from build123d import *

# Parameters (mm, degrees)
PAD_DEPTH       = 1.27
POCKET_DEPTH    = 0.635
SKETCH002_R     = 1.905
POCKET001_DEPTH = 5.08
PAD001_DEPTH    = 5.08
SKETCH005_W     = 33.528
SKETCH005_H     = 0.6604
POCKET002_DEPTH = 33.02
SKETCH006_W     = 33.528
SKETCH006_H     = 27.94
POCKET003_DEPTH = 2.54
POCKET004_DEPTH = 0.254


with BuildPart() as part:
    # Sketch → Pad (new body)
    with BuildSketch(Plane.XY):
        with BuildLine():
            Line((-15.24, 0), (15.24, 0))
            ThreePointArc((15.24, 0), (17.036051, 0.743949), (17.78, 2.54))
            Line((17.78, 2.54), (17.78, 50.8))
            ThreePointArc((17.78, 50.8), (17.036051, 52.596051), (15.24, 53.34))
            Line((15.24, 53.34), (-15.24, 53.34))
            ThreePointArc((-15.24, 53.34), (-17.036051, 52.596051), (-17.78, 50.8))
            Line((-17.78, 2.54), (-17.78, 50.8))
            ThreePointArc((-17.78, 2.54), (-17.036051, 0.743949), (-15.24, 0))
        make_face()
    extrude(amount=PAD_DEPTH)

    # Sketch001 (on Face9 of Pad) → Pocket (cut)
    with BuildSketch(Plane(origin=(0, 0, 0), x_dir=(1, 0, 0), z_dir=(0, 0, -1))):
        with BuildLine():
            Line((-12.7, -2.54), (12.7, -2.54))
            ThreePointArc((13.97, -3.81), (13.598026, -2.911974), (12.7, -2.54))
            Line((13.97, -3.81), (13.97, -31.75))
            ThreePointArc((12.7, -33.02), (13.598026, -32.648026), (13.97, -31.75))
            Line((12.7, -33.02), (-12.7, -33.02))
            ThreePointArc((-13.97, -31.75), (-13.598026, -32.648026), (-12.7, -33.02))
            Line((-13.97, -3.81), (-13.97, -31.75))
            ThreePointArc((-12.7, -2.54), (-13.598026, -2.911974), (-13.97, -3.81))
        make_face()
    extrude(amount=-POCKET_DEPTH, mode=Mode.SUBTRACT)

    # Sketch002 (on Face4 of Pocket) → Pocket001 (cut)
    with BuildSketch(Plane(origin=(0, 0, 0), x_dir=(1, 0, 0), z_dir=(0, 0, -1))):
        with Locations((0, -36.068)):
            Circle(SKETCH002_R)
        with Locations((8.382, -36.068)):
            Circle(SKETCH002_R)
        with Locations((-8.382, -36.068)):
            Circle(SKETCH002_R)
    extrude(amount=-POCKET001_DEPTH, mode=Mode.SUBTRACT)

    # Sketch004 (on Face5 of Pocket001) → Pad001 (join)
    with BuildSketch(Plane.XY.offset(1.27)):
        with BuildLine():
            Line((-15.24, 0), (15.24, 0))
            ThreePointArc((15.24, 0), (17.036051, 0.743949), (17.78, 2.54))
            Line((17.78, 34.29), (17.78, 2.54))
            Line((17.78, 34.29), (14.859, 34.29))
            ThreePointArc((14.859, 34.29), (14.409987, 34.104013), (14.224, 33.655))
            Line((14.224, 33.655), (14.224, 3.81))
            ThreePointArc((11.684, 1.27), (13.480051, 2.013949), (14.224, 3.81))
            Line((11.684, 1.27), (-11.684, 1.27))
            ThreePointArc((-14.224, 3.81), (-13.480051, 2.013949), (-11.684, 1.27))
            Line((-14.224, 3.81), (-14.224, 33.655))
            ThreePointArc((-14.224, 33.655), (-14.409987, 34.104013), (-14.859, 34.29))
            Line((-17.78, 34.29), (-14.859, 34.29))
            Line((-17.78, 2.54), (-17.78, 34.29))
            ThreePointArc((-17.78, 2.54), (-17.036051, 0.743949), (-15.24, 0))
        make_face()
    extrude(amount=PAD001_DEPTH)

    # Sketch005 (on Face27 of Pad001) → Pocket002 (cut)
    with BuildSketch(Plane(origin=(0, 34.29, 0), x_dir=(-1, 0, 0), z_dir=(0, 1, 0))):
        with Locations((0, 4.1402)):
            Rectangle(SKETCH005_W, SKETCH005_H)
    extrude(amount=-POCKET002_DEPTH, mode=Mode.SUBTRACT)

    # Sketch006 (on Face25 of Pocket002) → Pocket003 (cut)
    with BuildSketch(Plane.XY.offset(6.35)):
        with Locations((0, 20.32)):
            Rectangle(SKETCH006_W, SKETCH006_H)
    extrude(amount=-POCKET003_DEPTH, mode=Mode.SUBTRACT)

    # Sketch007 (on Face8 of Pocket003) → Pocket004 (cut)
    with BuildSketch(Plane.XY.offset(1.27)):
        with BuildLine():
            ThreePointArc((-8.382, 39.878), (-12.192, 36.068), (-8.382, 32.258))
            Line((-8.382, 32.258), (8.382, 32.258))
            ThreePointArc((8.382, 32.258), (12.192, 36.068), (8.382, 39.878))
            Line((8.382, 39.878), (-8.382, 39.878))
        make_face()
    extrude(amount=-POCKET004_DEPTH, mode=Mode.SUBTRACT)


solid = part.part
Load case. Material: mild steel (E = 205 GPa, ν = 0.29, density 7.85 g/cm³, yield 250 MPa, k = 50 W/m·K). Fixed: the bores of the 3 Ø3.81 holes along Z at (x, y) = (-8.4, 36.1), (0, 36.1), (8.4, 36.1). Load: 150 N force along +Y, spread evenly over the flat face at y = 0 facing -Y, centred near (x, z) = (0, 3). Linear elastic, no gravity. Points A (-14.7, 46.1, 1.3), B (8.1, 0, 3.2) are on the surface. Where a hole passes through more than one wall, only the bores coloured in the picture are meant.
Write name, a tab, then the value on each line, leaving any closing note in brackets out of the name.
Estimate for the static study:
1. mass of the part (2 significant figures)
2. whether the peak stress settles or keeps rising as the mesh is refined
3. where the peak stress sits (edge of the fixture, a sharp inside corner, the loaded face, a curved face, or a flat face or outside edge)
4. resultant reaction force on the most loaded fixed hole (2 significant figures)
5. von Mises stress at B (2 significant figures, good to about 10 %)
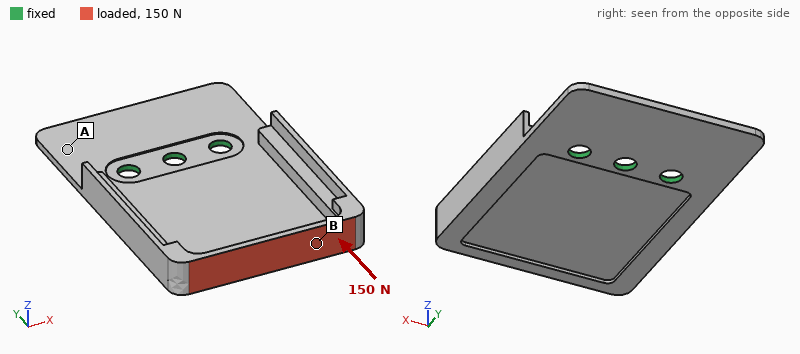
mass of the part	22 g
whether the peak stress settles or keeps rising as the mesh is refined	keeps rising
where the peak stress sits	a sharp inside corner
resultant reaction force on the most loaded fixed hole	52 N
von Mises stress at B	28 MPa
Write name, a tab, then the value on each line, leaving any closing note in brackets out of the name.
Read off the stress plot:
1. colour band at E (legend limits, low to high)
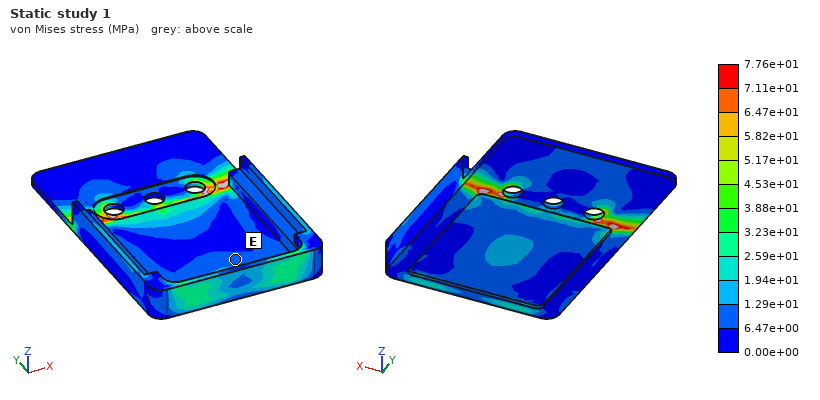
colour band at E	6.47e+00 to 1.29e+01 MPa
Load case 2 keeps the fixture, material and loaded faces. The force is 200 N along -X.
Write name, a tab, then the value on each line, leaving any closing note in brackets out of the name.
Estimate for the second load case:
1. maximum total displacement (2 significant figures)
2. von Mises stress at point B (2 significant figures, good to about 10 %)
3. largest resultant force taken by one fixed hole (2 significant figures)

maximum total displacement	84 µm
von Mises stress at point B	26 MPa
largest resultant force taken by one fixed hole	360 N
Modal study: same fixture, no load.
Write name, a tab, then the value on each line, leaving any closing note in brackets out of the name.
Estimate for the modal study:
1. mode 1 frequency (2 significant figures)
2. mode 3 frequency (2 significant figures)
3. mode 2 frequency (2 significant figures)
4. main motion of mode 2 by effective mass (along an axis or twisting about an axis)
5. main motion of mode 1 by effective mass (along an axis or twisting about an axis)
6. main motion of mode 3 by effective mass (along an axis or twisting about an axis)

mode 1 frequency	600 Hz
mode 3 frequency	3500 Hz
mode 2 frequency	1300 Hz
main motion of mode 2 by effective mass	twisting about Y
main motion of mode 1 by effective mass	along Z
main motion of mode 3 by effective mass	along Z
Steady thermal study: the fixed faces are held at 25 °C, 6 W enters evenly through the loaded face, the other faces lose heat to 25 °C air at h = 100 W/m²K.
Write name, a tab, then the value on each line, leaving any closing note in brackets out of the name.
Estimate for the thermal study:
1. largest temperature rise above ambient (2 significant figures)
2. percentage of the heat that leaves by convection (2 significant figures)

largest temperature rise above ambient	43 K
percentage of the heat that leaves by convection	87 %
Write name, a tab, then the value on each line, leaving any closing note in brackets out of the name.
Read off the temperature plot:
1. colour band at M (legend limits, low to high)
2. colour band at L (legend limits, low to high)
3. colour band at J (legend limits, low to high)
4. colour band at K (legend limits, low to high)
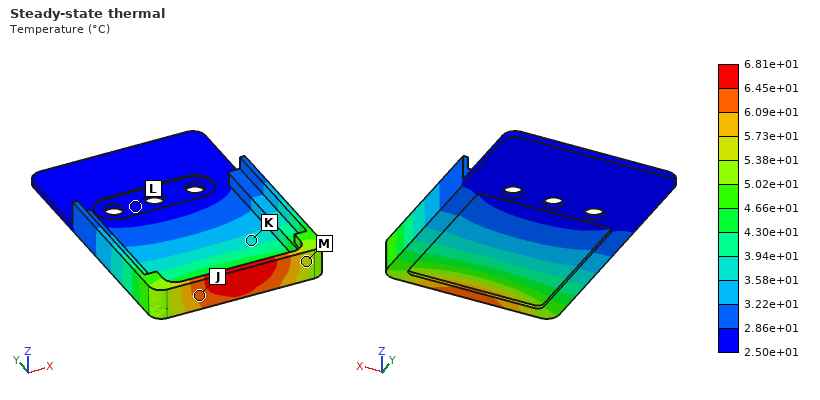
colour band at M	5.38e+01 to 5.73e+01 °C
colour band at L	2.50e+01 to 2.86e+01 °C
colour band at J	6.09e+01 to 6.45e+01 °C
colour band at K	3.58e+01 to 3.94e+01 °C
